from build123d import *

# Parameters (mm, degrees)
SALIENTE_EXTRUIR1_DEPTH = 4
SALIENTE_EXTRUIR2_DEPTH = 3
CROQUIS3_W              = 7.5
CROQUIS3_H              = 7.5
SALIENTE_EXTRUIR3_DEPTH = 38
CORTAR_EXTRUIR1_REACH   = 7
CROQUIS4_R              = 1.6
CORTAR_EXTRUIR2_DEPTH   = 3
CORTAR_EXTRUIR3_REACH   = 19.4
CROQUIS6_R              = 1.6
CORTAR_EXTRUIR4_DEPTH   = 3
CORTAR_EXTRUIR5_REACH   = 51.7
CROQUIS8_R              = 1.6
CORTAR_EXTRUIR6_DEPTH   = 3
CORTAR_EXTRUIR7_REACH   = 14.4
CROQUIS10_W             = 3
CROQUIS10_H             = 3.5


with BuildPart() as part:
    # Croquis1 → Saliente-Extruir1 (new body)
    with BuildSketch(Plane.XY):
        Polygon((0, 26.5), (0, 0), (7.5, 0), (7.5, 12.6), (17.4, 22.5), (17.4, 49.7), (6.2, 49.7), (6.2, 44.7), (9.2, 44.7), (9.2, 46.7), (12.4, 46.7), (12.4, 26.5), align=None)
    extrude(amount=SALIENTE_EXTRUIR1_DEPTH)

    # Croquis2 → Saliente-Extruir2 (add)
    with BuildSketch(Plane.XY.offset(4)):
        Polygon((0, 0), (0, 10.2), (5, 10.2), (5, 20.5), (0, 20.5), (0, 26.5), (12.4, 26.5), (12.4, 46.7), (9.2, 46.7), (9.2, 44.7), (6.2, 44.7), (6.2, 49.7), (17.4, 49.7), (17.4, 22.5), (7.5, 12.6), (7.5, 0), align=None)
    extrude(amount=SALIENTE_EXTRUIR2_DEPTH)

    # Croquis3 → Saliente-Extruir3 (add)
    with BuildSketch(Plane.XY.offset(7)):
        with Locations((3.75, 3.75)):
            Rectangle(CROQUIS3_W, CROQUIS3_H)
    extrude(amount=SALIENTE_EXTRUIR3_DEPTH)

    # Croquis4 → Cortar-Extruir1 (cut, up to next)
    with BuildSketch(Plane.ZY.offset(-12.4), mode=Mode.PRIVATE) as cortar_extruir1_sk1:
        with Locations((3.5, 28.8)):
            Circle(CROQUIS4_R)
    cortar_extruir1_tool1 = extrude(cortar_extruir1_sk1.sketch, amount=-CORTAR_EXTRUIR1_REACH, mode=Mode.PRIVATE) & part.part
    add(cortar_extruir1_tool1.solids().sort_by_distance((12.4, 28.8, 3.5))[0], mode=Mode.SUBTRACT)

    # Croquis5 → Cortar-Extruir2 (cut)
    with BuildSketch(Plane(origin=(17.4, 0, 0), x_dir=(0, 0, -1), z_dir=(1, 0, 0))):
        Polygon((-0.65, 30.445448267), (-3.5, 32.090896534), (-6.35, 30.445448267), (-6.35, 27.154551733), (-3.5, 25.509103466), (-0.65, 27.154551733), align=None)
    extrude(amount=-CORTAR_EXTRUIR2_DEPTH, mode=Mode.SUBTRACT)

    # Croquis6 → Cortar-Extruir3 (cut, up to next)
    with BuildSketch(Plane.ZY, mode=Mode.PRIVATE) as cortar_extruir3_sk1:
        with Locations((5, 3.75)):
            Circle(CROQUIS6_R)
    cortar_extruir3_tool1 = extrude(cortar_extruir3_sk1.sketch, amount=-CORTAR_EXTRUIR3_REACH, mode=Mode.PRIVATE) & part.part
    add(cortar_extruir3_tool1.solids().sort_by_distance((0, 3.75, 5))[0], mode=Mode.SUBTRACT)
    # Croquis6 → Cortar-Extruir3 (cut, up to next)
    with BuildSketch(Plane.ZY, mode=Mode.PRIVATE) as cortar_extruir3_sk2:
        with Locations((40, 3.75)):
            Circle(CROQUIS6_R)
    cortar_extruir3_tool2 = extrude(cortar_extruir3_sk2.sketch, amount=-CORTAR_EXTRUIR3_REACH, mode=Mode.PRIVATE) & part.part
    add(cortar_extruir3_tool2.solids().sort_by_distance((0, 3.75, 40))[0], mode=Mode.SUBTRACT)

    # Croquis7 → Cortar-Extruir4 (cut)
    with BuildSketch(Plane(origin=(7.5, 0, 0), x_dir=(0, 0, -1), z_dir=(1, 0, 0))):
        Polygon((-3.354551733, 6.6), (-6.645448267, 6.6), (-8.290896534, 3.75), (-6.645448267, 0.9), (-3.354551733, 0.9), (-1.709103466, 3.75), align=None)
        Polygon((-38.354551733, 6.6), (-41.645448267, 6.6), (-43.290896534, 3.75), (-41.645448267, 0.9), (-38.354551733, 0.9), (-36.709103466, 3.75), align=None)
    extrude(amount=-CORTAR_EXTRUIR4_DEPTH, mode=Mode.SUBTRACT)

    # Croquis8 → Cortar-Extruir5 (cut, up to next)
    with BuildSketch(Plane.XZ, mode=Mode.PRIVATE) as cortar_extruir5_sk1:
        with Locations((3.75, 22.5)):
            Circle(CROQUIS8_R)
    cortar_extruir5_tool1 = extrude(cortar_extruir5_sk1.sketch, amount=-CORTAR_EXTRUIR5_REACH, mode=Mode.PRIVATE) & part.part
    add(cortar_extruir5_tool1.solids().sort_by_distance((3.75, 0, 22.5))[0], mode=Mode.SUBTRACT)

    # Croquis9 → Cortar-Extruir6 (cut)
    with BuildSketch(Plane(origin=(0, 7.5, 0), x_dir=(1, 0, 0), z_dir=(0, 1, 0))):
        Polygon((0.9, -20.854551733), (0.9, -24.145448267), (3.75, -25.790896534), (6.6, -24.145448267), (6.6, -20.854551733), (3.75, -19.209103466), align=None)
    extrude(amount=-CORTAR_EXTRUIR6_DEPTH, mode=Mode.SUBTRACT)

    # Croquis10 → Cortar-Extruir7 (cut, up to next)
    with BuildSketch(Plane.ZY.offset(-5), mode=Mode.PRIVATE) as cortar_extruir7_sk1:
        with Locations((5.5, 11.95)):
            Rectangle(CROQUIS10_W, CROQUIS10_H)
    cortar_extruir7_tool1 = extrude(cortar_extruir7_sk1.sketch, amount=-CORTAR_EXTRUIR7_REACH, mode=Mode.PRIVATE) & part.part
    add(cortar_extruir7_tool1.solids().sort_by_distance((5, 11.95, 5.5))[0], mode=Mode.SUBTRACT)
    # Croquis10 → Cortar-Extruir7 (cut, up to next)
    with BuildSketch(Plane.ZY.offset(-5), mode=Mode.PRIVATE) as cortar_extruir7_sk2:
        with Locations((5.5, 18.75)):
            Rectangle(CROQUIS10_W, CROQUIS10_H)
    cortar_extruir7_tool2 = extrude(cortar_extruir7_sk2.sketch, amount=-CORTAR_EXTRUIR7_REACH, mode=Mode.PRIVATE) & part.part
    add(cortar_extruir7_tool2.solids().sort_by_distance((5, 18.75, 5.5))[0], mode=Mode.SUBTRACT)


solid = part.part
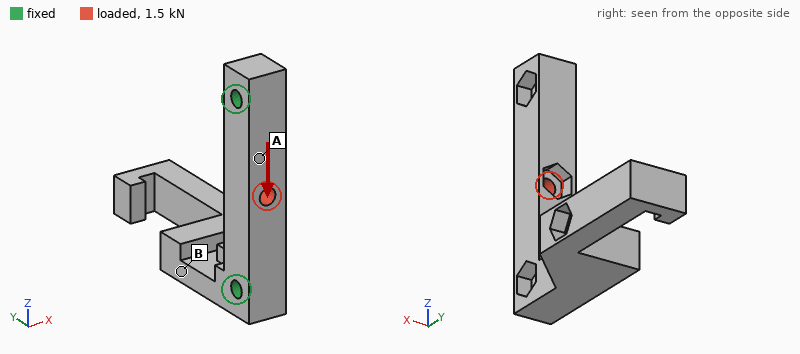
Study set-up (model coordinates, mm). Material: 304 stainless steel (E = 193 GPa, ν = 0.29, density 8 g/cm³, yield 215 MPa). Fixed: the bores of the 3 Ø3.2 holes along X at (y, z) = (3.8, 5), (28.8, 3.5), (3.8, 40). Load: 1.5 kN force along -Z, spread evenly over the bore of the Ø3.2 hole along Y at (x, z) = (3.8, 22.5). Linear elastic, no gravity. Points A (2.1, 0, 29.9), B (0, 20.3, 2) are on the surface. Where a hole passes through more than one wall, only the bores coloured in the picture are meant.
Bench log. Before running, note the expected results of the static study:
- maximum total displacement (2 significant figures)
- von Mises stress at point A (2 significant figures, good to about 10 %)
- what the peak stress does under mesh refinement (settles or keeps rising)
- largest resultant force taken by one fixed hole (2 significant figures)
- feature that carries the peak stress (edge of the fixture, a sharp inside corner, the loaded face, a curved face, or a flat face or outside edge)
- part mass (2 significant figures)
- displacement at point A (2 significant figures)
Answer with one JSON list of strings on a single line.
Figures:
["1.9 µm", "24 MPa", "keeps rising", "750 N", "edge of the fixture", "35 g", "1.00 µm"]
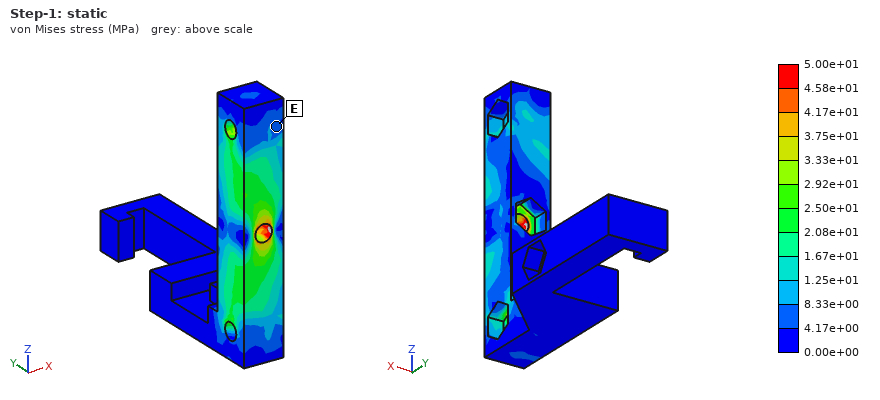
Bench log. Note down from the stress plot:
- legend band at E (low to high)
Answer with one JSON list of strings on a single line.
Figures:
["4.17e+00 to 8.33e+00 MPa"]
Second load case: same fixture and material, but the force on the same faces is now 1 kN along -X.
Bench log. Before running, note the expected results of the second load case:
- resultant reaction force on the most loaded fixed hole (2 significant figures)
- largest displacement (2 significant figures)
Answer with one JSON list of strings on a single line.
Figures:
["620 N", "11 µm"]
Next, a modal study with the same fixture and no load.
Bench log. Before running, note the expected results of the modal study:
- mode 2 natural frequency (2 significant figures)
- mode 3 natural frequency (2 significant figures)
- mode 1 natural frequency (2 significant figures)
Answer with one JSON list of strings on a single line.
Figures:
["6700 Hz", "14 kHz", "4500 Hz"]
